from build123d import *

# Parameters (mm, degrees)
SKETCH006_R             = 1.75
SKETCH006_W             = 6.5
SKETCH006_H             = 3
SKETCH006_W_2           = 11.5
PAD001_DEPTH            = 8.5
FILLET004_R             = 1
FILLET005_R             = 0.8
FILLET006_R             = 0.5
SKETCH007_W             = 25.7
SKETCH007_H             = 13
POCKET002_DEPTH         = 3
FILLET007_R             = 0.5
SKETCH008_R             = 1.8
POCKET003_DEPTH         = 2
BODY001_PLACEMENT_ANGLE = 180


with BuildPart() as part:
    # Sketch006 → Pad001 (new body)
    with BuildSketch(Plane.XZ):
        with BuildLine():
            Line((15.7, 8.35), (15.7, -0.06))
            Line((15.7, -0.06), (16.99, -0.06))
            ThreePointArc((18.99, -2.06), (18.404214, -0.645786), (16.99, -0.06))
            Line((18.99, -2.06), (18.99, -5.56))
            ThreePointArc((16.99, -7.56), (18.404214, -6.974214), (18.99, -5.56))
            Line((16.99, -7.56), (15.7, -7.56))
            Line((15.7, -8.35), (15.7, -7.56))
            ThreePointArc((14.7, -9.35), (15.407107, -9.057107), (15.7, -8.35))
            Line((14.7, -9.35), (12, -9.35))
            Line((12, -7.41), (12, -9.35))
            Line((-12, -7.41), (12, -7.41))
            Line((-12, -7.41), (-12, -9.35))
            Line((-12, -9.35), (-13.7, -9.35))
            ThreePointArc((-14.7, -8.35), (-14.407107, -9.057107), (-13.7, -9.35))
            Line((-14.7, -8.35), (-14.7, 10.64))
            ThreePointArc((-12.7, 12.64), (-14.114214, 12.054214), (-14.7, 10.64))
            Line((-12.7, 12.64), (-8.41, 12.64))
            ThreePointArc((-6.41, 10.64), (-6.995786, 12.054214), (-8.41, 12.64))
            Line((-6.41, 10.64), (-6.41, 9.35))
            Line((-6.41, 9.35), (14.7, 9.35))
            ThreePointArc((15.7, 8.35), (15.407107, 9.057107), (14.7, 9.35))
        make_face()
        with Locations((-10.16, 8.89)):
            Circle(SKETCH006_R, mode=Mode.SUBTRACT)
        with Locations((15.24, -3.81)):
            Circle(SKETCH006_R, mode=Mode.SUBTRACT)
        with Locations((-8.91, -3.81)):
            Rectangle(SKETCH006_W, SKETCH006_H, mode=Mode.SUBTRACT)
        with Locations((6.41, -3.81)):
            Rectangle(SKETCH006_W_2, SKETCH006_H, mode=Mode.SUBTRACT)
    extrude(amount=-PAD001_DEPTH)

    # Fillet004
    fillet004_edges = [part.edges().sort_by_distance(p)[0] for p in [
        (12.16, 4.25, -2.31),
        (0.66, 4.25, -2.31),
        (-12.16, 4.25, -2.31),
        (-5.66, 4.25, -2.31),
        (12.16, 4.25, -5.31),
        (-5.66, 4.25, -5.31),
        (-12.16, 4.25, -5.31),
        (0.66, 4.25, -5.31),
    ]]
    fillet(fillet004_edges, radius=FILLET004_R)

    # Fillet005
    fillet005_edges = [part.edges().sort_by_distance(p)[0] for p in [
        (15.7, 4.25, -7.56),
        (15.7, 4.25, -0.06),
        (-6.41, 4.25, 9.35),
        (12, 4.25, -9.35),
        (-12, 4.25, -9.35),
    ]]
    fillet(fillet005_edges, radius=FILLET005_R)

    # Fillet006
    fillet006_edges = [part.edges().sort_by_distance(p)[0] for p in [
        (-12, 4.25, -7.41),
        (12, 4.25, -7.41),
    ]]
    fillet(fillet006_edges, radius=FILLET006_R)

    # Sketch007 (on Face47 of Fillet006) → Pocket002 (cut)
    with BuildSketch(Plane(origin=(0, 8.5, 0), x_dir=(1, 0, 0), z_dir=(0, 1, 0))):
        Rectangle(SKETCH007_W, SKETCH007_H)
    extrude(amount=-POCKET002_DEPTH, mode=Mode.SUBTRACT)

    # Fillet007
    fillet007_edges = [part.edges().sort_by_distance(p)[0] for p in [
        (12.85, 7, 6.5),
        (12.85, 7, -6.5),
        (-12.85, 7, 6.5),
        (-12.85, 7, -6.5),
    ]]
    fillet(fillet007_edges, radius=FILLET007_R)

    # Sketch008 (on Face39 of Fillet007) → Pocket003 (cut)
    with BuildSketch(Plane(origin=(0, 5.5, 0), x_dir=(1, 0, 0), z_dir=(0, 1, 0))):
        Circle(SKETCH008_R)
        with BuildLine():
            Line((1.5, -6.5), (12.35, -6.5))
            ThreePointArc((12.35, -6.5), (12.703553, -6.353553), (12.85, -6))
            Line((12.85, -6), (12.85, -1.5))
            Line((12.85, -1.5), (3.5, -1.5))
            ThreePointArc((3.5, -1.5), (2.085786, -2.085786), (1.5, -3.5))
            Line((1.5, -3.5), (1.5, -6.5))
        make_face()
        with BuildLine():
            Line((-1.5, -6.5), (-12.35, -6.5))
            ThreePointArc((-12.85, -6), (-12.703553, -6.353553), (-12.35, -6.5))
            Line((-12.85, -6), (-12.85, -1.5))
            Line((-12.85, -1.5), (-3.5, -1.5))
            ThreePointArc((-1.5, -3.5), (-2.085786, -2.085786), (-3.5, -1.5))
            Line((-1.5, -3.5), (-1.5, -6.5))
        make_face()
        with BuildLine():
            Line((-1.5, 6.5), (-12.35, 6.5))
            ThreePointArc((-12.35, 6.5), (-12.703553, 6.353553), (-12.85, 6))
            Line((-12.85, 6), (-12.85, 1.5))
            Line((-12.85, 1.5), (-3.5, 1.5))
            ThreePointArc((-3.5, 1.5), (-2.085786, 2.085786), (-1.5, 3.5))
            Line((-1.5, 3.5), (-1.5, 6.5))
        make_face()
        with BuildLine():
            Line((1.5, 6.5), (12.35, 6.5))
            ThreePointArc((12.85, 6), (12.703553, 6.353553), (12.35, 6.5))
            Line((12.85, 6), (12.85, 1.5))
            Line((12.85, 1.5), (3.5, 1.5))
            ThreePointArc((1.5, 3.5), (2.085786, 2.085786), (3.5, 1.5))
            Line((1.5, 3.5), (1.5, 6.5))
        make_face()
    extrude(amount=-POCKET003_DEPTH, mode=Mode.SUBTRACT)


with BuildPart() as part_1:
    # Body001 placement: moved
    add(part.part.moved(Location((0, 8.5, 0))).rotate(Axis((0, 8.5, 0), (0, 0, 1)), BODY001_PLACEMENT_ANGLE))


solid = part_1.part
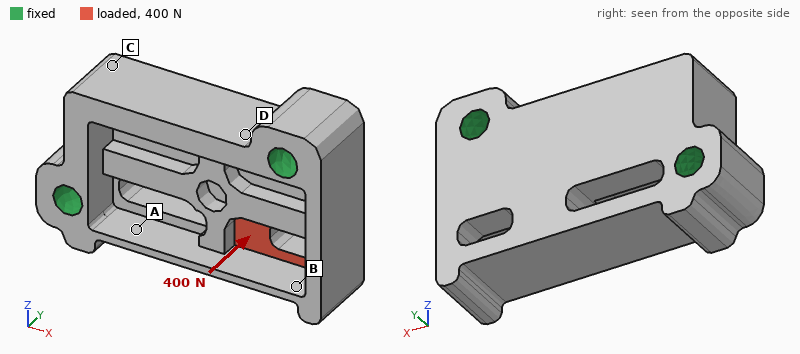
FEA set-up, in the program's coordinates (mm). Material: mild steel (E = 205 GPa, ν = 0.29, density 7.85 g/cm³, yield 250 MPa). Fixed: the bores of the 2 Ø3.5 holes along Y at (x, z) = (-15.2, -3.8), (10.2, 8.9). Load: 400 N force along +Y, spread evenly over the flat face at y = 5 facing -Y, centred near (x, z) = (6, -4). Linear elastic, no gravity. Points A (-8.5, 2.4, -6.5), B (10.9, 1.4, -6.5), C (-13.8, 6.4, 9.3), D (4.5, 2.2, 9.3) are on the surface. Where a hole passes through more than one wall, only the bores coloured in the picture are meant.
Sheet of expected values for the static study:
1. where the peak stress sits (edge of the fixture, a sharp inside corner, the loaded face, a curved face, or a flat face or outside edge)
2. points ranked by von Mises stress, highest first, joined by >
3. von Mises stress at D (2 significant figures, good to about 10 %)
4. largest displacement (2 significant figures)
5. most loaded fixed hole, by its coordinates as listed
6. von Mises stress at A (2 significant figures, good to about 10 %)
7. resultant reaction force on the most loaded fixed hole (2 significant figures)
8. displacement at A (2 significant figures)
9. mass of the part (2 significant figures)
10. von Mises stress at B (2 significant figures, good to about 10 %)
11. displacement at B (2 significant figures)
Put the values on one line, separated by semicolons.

a curved face; A > B > D > C; 9.6 MPa; 9.1 µm; (10.2, 8.9); 25 MPa; 290 N; 1.8 µm; 24 g; 18 MPa; 7.5 µm
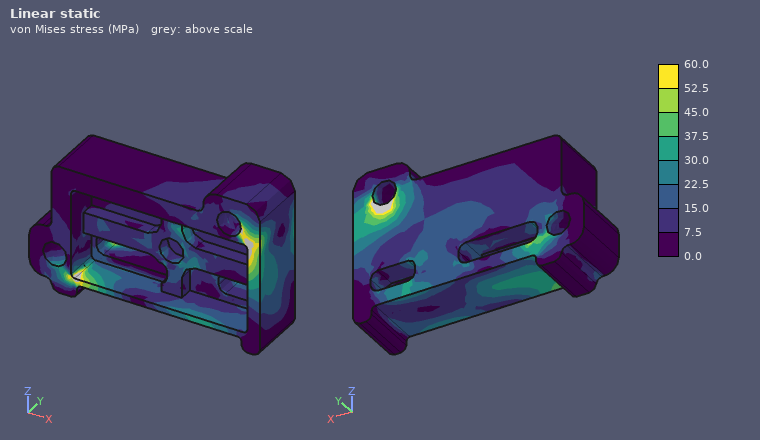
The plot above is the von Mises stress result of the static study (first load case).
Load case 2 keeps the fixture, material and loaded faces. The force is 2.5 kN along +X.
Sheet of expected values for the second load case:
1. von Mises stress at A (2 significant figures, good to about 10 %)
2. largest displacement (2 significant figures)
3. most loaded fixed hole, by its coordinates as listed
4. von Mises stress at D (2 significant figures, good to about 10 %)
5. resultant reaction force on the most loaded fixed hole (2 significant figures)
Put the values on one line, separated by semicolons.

86 MPa; 11 µm; (-15.2, -3.8); 21 MPa; 1.5 kN
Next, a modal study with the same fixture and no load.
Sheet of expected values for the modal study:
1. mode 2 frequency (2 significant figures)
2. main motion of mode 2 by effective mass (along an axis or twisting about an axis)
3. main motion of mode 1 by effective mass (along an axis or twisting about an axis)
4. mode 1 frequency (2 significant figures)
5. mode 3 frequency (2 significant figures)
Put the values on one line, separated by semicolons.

28 kHz; along Y; along Y; 17 kHz; 31 kHz
